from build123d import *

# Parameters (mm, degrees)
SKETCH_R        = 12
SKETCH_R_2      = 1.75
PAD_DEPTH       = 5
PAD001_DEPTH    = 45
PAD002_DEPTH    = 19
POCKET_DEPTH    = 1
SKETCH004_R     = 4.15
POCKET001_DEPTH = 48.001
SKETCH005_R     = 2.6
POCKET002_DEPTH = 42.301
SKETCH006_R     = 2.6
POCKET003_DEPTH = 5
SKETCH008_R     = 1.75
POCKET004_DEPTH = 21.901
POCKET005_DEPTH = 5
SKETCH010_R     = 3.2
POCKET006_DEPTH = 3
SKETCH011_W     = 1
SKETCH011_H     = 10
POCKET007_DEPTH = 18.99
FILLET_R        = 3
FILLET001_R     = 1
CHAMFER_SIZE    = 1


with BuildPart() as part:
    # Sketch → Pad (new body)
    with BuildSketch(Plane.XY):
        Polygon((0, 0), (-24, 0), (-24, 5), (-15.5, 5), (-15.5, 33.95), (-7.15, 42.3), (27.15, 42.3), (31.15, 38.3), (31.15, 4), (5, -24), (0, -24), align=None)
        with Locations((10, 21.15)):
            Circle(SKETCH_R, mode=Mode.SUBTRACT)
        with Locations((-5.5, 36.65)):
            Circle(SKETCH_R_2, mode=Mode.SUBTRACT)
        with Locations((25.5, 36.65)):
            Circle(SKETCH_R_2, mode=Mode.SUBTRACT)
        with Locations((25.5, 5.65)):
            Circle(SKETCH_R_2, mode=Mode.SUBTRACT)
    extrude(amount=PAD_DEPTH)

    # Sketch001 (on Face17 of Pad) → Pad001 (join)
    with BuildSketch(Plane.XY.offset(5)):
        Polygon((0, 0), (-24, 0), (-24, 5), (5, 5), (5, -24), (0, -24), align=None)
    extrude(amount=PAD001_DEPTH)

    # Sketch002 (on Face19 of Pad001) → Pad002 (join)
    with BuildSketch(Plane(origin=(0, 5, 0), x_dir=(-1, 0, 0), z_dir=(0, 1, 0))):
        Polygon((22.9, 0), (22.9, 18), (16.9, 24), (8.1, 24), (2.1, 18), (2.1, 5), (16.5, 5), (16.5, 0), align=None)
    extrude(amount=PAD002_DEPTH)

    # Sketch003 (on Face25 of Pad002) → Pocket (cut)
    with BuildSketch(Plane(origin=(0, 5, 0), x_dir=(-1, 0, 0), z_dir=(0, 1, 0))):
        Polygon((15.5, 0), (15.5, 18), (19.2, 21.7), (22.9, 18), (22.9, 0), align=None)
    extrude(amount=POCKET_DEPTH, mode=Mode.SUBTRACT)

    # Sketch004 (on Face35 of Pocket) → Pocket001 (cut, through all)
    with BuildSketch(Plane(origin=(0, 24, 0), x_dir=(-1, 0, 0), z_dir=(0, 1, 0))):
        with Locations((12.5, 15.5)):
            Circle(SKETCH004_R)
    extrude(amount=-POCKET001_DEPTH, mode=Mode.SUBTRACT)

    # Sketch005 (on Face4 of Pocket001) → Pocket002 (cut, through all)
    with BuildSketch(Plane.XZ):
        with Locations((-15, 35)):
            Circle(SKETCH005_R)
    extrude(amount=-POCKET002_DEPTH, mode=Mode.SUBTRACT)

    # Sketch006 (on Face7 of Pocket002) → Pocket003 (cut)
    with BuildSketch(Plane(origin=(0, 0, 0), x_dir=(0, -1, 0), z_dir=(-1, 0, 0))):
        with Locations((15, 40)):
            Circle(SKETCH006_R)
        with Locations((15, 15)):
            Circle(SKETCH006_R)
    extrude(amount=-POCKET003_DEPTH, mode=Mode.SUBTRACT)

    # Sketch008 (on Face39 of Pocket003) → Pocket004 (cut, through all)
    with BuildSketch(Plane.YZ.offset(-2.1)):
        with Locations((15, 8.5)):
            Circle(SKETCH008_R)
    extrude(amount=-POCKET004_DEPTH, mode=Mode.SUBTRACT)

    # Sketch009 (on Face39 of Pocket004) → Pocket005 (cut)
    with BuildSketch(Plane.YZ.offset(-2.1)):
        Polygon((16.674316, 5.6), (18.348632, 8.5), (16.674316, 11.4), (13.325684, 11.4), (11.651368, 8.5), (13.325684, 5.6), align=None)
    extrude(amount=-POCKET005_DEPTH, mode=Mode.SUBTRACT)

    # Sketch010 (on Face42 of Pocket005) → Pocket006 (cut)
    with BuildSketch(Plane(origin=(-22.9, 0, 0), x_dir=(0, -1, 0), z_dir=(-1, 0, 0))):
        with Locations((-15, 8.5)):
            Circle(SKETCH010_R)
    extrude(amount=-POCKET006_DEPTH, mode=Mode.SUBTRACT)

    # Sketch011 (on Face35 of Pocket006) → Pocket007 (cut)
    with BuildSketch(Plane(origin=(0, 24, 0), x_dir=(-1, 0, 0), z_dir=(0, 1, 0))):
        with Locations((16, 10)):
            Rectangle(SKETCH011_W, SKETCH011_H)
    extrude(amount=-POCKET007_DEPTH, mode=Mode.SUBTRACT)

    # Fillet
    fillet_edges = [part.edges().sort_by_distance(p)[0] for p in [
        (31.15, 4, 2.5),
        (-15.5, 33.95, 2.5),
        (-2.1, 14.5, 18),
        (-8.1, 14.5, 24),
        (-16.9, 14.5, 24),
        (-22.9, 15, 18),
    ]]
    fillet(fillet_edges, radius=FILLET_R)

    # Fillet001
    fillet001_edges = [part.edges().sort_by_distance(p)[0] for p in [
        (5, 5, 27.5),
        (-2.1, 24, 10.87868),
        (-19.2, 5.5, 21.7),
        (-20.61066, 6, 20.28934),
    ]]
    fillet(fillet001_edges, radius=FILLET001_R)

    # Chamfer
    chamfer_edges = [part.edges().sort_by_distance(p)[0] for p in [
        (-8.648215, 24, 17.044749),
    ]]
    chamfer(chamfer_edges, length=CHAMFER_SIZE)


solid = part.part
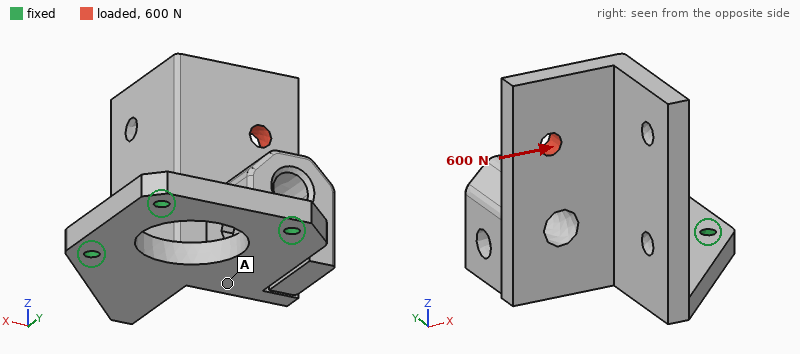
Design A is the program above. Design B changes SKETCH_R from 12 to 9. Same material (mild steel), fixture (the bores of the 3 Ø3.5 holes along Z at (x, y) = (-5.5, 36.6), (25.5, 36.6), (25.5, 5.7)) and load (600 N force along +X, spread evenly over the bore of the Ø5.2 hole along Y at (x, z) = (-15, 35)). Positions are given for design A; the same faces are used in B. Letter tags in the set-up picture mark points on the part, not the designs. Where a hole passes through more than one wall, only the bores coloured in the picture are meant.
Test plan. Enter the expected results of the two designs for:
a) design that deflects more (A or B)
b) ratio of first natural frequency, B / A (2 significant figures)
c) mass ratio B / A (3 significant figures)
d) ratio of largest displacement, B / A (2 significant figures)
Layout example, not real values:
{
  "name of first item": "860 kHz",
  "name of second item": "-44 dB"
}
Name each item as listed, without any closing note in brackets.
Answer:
{
  "design that deflects more": "A",
  "ratio of first natural frequency, B / A": "1.1",
  "mass ratio B / A": "1.04",
  "ratio of largest displacement, B / A": "0.84"
}
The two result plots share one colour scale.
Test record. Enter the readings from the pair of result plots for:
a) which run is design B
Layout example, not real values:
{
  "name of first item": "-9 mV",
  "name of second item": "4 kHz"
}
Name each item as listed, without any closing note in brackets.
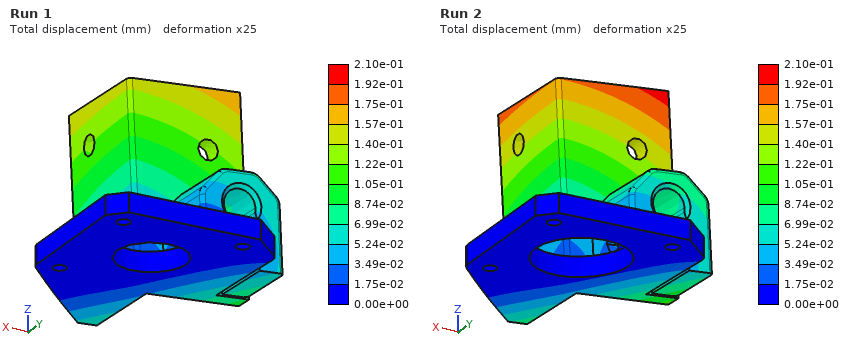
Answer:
{
  "which run is design B": "Run 1"
}
